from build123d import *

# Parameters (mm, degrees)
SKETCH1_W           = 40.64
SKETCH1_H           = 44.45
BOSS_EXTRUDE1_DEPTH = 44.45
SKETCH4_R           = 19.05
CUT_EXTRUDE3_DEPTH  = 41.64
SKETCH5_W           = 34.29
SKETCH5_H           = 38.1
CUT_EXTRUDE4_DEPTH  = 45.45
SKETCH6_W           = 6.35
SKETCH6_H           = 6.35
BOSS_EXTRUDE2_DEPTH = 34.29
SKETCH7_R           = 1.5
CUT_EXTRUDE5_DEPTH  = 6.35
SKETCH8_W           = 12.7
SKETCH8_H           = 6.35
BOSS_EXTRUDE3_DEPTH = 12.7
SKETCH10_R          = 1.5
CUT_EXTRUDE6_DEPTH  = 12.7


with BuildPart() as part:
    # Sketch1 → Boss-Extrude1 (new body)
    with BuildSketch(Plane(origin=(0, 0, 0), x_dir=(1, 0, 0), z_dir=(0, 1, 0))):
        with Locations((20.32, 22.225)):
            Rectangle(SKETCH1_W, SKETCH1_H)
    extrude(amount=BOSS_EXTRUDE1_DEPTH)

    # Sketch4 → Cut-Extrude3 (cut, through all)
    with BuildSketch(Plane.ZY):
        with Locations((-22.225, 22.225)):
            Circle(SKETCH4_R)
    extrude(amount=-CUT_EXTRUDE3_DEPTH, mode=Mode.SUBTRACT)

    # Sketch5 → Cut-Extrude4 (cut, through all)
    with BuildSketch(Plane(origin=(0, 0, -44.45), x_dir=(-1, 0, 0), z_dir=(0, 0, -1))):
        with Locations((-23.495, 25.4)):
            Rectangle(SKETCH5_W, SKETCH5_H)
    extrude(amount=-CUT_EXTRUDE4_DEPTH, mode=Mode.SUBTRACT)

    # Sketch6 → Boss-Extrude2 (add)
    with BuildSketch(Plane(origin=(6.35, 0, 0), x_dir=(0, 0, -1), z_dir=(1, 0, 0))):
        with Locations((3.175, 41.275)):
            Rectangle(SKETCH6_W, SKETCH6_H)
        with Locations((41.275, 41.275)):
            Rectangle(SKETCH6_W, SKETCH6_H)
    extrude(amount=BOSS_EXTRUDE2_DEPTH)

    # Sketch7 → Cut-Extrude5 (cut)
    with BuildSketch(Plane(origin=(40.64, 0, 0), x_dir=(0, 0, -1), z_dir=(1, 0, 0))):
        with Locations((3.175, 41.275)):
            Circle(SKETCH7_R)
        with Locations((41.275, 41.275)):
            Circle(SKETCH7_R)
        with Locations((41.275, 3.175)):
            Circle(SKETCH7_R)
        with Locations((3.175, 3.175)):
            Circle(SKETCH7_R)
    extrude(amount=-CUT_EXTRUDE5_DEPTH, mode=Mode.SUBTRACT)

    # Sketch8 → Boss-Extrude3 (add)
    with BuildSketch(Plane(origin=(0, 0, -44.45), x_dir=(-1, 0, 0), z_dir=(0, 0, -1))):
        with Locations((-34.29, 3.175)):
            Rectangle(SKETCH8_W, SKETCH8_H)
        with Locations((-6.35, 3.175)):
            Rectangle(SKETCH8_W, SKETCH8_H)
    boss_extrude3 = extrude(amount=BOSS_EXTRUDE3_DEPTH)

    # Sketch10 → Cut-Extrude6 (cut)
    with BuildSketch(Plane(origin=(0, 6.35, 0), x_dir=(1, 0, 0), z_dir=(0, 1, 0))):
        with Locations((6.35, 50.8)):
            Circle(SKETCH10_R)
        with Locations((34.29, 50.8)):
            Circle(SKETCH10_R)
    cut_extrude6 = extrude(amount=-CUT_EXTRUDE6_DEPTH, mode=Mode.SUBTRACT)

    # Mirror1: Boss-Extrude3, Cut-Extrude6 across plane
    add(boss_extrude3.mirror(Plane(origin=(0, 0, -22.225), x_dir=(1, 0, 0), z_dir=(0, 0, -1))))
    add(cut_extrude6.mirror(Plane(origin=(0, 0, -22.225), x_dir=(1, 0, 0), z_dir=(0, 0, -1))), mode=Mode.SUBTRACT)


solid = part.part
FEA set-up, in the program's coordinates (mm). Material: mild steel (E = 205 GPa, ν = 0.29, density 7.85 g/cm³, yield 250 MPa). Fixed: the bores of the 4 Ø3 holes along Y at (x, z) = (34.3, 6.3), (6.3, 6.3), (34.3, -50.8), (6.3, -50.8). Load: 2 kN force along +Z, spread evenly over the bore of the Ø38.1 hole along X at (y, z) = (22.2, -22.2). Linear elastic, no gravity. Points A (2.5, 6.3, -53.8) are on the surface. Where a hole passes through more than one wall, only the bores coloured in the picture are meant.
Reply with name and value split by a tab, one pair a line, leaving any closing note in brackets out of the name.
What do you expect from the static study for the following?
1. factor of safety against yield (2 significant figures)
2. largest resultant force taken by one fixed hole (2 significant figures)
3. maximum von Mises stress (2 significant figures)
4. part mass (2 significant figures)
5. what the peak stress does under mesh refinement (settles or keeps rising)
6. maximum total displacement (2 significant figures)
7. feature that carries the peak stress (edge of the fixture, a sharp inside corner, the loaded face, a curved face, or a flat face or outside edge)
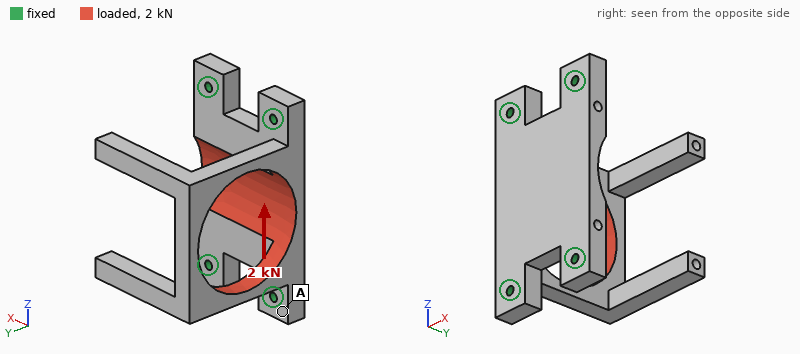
factor of safety against yield	2.6
largest resultant force taken by one fixed hole	730 N
maximum von Mises stress	97 MPa
part mass	160 g
what the peak stress does under mesh refinement	settles
maximum total displacement	51 µm
feature that carries the peak stress	the loaded face
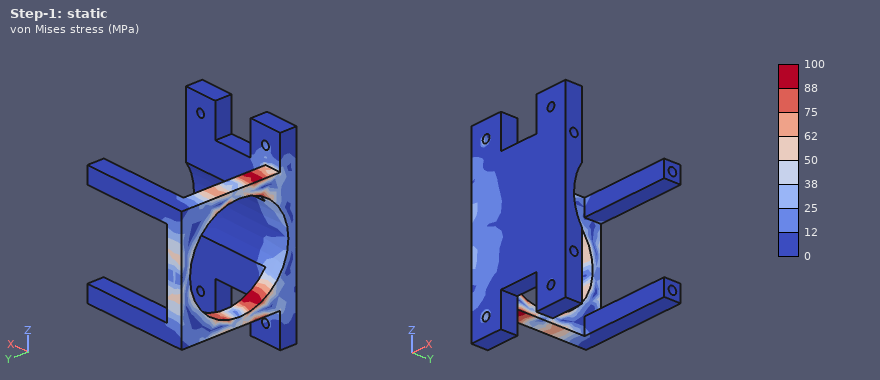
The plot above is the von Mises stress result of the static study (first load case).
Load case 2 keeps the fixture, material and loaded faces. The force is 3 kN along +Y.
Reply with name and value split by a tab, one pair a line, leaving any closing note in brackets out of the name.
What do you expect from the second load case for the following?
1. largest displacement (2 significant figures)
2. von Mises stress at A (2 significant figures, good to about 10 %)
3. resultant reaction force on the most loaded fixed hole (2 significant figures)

largest displacement	23 µm
von Mises stress at A	23 MPa
resultant reaction force on the most loaded fixed hole	1.3 kN
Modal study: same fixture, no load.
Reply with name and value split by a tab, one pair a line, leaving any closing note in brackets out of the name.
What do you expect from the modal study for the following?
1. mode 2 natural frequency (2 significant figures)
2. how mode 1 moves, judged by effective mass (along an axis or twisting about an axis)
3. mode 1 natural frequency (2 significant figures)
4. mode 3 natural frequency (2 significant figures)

mode 2 natural frequency	1300 Hz
how mode 1 moves, judged by effective mass	along X
mode 1 natural frequency	1000 Hz
mode 3 natural frequency	2200 Hz
